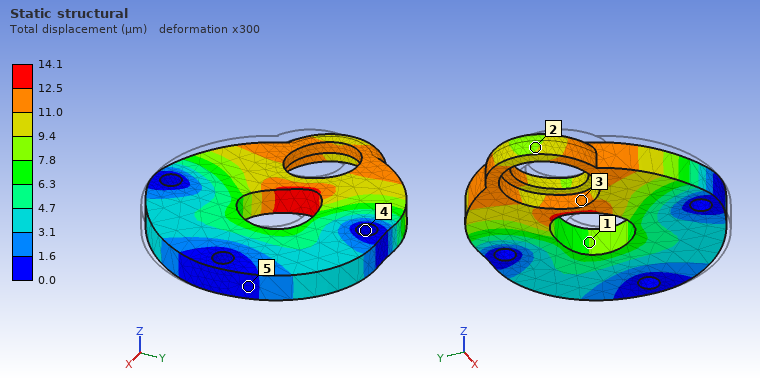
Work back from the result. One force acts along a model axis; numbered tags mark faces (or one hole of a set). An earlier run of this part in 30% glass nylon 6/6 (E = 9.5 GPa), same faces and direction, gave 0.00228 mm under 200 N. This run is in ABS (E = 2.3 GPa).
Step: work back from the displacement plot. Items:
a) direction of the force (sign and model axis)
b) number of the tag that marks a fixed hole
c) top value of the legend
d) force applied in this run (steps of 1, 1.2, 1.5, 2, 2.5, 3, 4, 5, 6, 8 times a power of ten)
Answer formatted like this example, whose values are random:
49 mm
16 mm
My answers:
+Y
4
14.1 µm
300 N
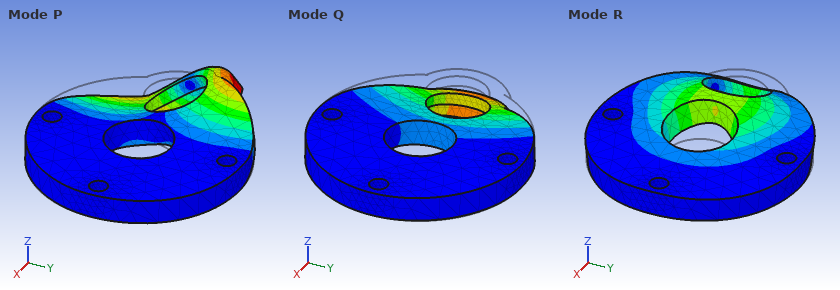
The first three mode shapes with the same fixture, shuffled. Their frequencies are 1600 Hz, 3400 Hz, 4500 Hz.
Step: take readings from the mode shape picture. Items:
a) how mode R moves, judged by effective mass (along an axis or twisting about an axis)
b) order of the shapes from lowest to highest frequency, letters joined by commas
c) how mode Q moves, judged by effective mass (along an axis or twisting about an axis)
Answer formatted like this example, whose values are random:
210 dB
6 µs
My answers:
along Z
Q, P, R
along Z
